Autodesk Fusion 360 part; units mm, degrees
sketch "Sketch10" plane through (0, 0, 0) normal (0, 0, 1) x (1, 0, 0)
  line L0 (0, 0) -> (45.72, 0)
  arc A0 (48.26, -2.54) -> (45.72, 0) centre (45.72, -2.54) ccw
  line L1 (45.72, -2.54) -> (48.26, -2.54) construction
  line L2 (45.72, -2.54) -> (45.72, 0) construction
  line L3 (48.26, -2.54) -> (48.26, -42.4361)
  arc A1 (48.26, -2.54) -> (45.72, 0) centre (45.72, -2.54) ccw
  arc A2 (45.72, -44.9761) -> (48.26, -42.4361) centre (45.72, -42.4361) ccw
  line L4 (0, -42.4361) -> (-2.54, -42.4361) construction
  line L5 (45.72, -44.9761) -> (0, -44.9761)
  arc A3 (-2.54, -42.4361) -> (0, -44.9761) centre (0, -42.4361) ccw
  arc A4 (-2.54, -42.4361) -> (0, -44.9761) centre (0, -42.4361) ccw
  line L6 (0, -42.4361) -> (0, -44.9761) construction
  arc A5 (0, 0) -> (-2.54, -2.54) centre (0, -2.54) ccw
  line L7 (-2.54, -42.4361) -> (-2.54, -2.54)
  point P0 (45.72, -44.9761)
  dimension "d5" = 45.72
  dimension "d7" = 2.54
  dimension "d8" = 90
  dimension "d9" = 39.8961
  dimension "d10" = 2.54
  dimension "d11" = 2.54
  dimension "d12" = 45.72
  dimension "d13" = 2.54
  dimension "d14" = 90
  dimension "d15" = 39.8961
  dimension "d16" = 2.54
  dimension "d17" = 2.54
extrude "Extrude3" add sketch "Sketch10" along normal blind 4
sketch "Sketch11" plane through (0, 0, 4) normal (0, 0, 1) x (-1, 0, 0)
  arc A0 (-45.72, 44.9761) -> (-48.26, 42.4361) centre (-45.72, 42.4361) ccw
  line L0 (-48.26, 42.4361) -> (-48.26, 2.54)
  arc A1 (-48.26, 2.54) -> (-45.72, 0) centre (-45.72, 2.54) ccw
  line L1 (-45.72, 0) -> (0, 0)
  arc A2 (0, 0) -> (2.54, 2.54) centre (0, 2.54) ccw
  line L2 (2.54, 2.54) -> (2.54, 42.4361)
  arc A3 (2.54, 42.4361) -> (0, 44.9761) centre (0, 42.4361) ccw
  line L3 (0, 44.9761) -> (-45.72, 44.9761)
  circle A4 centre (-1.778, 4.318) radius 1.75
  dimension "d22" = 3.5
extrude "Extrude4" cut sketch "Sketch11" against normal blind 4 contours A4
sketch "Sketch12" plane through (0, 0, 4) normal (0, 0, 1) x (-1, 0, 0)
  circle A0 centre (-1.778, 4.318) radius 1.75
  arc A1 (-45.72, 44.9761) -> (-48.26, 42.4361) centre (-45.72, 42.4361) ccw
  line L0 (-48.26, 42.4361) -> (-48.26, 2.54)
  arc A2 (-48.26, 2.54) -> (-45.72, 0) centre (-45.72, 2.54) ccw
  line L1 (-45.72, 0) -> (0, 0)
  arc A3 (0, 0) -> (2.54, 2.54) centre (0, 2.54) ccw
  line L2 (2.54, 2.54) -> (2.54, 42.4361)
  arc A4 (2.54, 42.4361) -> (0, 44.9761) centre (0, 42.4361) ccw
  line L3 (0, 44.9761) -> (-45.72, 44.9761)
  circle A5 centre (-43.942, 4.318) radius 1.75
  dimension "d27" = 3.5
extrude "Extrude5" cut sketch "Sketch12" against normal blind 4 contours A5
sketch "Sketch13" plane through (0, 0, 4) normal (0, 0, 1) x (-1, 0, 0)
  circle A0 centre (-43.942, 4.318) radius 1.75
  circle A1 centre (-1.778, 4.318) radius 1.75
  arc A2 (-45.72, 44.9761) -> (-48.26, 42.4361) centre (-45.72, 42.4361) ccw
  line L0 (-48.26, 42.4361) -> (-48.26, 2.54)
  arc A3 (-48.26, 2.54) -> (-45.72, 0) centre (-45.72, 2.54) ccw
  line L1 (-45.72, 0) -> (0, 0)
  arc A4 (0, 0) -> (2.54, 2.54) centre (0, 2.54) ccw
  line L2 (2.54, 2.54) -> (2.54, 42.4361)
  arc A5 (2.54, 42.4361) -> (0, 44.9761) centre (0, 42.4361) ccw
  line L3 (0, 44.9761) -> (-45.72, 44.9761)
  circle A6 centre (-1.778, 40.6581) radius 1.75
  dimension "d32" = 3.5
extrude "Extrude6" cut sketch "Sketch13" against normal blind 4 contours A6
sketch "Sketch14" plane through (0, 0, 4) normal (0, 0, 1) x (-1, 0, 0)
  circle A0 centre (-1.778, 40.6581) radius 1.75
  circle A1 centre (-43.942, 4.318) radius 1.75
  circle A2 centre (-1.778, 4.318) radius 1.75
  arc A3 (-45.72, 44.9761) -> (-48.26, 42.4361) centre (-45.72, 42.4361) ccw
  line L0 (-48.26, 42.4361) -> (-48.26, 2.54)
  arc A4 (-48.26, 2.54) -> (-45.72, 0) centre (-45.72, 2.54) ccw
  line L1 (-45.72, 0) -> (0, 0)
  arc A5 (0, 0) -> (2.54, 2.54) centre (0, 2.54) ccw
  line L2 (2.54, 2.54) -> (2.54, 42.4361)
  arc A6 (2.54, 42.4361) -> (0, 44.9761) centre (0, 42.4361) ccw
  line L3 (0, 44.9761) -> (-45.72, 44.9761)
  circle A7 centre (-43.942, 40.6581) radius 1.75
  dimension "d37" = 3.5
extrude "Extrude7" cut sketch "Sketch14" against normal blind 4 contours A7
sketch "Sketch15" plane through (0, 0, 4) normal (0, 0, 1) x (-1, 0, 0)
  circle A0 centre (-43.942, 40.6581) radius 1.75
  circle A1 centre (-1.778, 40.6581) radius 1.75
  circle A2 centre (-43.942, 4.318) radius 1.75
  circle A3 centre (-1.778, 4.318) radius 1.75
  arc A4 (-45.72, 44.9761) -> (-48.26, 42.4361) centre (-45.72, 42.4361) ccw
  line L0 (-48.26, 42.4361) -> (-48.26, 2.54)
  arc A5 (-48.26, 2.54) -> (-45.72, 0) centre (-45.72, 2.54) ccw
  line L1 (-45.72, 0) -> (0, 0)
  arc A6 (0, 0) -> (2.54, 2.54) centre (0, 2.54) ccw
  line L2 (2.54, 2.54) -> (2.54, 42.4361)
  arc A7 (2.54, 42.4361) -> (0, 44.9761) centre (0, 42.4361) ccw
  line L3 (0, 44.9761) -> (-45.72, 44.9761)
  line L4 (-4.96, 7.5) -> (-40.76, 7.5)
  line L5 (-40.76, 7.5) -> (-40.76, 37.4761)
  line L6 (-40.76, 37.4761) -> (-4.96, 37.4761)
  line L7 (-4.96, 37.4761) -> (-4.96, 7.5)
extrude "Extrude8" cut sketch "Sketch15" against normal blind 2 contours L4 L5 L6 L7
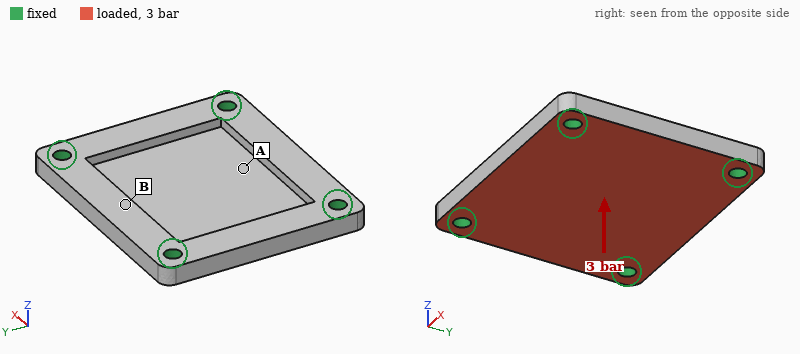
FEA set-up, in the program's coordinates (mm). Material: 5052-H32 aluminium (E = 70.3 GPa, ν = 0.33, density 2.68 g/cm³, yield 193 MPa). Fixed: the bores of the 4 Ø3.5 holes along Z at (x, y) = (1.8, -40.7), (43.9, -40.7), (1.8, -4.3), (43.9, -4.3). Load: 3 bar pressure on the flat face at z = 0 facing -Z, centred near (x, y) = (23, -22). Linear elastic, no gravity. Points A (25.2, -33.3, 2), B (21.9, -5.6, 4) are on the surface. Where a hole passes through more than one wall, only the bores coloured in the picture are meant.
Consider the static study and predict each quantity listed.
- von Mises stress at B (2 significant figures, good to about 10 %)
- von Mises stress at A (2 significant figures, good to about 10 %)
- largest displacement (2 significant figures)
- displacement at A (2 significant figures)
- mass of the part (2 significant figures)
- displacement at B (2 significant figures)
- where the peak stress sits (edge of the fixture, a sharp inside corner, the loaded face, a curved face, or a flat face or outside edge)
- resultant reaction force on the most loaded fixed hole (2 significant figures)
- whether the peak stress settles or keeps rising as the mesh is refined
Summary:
17 MPa
7.4 MPa
30 µm
21 µm
18 g
13 µm
edge of the fixture
190 N
keeps rising
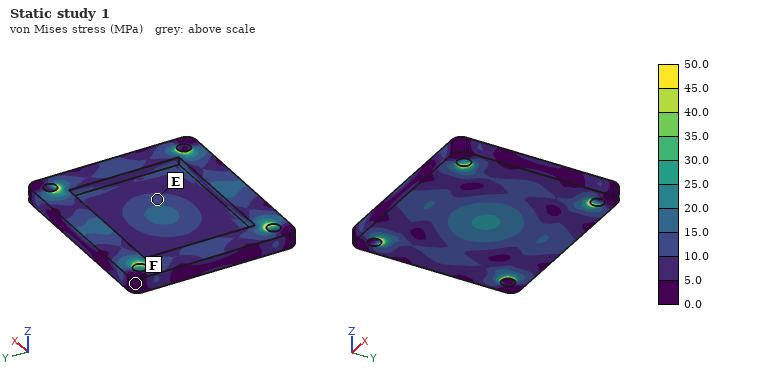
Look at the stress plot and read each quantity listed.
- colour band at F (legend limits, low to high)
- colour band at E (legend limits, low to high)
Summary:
0.0 to 5.0 MPa
10.0 to 15.0 MPa
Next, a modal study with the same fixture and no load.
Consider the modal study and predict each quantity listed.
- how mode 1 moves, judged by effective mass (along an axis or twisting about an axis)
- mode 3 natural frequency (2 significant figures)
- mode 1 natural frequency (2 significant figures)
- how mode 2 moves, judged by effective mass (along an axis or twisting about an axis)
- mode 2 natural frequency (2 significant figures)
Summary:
along Z
14 kHz
8400 Hz
twisting about X
12 kHz
